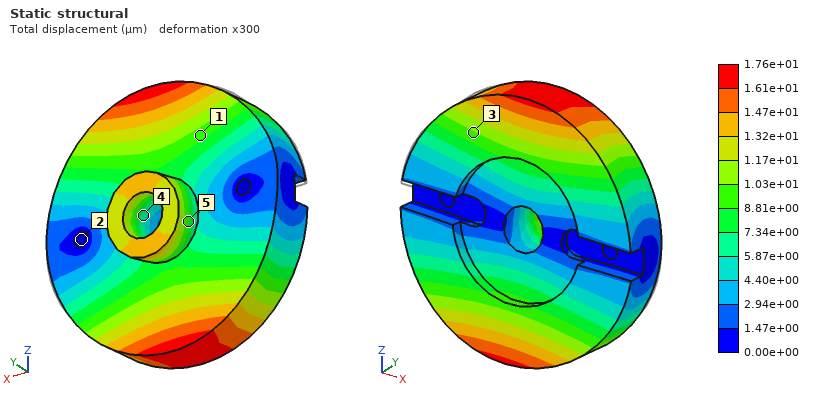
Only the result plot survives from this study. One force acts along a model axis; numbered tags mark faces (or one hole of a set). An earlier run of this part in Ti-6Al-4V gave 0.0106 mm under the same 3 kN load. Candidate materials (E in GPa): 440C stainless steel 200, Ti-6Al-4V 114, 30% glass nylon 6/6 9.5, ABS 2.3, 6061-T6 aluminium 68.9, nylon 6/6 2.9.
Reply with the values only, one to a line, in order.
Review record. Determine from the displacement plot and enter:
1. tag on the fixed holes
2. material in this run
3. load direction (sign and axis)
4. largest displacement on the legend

2
6061-T6 aluminium
-Z
1.76e+01 µm
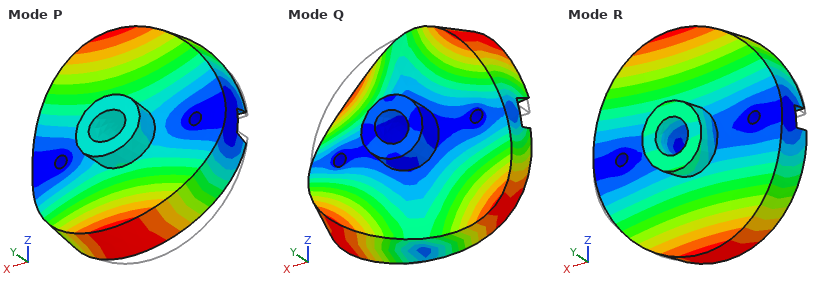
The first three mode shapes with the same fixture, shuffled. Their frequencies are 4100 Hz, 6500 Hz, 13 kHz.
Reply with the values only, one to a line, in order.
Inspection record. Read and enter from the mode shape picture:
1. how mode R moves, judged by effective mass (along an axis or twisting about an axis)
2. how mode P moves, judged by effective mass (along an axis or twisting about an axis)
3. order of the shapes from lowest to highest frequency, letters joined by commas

twisting about X
along Y
R, P, Q
